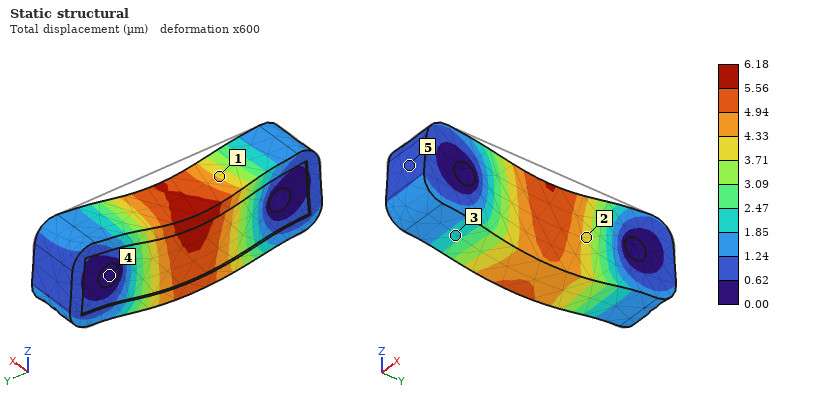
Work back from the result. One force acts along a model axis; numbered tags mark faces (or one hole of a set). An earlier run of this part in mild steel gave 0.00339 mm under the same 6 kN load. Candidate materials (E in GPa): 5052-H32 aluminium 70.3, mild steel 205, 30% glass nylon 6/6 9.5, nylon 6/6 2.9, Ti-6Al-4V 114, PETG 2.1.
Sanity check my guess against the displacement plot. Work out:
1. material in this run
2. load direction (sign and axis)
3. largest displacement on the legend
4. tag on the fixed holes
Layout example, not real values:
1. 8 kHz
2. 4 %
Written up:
1. Ti-6Al-4V
2. -Z
3. 6.18 µm
4. 4
